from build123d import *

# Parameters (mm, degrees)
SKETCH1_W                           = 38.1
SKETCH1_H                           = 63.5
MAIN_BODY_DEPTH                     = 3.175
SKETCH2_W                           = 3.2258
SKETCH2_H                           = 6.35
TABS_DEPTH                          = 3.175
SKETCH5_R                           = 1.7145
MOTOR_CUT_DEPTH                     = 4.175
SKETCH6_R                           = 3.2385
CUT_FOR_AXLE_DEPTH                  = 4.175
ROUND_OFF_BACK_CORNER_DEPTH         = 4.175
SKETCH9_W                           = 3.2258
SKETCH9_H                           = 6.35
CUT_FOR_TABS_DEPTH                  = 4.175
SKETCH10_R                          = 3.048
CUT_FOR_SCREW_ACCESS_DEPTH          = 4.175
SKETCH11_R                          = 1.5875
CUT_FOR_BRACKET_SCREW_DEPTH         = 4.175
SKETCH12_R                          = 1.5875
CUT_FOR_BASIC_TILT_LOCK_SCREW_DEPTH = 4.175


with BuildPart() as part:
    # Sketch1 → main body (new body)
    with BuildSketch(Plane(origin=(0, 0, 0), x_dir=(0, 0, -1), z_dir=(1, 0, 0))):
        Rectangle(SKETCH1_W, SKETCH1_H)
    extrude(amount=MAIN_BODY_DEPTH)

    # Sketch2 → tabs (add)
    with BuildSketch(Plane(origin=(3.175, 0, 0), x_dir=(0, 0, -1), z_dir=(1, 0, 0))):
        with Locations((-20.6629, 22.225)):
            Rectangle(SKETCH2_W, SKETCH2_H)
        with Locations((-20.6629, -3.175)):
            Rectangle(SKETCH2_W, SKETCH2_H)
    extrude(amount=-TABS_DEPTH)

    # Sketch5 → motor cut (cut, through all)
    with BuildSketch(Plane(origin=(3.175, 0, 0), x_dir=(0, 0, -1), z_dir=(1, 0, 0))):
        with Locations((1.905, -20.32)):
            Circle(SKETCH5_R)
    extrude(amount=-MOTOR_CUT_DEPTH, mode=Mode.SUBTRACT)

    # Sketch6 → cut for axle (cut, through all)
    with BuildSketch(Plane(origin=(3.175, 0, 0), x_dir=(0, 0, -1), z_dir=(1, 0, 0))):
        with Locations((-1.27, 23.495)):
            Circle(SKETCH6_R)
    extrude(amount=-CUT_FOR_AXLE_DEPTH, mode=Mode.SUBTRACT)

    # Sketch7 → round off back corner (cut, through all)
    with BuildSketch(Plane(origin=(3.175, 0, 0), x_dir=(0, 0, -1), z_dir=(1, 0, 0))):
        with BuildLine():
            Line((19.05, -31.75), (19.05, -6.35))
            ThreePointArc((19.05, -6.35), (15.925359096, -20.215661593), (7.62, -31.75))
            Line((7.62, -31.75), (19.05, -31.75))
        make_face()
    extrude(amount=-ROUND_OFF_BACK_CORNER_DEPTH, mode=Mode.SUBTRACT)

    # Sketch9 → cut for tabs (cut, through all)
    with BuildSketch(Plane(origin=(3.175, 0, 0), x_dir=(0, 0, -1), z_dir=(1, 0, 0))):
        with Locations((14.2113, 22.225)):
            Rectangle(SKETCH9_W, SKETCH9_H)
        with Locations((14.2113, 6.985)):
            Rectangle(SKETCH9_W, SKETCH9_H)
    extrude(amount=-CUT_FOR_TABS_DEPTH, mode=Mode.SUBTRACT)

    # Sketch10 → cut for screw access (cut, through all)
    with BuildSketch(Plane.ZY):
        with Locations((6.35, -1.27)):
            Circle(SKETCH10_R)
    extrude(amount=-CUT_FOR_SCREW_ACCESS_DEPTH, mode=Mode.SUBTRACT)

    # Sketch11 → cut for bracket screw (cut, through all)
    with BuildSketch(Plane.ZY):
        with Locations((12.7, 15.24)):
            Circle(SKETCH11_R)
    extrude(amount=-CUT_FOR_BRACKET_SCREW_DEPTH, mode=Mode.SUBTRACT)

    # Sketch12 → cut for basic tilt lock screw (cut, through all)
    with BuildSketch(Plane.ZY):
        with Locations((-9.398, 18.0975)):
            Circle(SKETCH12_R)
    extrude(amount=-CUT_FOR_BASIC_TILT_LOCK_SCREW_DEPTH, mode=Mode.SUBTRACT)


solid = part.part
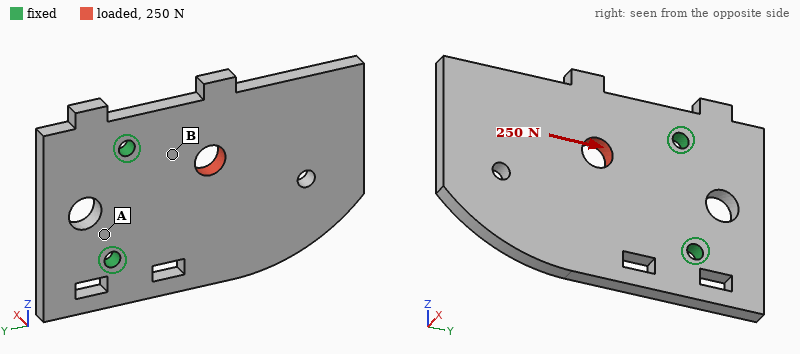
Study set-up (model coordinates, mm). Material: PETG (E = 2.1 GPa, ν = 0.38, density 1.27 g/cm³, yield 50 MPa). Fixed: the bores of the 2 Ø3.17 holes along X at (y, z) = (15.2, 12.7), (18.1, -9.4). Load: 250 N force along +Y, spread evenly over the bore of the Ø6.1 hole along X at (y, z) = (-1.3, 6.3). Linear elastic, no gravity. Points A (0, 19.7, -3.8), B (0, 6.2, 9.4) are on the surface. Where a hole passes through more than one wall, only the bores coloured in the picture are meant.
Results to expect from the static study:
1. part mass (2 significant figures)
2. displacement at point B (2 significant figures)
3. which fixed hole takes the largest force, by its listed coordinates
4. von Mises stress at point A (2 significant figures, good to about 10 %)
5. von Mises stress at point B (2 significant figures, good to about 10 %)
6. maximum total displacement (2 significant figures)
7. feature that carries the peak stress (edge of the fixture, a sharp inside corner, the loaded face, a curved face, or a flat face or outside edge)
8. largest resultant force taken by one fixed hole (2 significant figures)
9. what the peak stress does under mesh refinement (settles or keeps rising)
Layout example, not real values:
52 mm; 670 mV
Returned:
9.0 g; 21 µm; (15.2, 12.7); 1.0 MPa; 4.4 MPa; 50 µm; edge of the fixture; 180 N; keeps rising
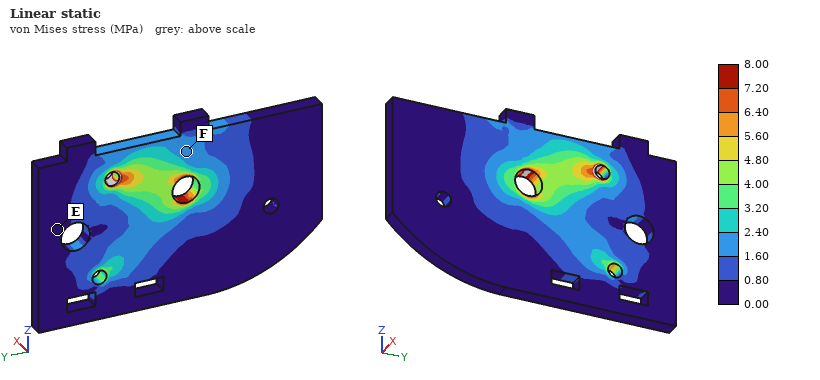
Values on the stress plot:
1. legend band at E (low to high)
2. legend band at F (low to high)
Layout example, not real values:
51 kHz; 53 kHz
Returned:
0.00 to 0.80 MPa; 1.60 to 2.40 MPa
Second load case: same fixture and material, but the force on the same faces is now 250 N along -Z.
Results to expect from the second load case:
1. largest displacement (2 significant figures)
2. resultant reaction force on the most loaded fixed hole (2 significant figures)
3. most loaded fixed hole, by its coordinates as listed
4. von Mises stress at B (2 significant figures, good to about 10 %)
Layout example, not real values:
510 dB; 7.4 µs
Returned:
0.17 mm; 240 N; (15.2, 12.7); 5.6 MPa
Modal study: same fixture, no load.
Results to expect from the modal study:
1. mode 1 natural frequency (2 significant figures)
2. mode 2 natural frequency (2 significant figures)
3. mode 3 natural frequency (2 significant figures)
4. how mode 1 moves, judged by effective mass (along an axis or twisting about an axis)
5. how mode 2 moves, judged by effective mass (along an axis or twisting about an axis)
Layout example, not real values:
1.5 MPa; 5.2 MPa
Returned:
290 Hz; 870 Hz; 1700 Hz; along X; twisting about Y
